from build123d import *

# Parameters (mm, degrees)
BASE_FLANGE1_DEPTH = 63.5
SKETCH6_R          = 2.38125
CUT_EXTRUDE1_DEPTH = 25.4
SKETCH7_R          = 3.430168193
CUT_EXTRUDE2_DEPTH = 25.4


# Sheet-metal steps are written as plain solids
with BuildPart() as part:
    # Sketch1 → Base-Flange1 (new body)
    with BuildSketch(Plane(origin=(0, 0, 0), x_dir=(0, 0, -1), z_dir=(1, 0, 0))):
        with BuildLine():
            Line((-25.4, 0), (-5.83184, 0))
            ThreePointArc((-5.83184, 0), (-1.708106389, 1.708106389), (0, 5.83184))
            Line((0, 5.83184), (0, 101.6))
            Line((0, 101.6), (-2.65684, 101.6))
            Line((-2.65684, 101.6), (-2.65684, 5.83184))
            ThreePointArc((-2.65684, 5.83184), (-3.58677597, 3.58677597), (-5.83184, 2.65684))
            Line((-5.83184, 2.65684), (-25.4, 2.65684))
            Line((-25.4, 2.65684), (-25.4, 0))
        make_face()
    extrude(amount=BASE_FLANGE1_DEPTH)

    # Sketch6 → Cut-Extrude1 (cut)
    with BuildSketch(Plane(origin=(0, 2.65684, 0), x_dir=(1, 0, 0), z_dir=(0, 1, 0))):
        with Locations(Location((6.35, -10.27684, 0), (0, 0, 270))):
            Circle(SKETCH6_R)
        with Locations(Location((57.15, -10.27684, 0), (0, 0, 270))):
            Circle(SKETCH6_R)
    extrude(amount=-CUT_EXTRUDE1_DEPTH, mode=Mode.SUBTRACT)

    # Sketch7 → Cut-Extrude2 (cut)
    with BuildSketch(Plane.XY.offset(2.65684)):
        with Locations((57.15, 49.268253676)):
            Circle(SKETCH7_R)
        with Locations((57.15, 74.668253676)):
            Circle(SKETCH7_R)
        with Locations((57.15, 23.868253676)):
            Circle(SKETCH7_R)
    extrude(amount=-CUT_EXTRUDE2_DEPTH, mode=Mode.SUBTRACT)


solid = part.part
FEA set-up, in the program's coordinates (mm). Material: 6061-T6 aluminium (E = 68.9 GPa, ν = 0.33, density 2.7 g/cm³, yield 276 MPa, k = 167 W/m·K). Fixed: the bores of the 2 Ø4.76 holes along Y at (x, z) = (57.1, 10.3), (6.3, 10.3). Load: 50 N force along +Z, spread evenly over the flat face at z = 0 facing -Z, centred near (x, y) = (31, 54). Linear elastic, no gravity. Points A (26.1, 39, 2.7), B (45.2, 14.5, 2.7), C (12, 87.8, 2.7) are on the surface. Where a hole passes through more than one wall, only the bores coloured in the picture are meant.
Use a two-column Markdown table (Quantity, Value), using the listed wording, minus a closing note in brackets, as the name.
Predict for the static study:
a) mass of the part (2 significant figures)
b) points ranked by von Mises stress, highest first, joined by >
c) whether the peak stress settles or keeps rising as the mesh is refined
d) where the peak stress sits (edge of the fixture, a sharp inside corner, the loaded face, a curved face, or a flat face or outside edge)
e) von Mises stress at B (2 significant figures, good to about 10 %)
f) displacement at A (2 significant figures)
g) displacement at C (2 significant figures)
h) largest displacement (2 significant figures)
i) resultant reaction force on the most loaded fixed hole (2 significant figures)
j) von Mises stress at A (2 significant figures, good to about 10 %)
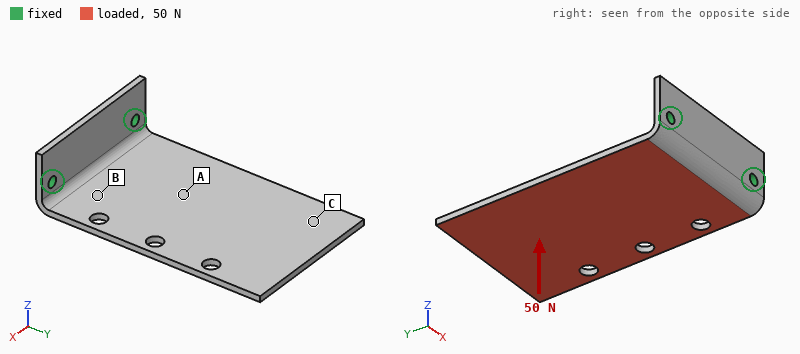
| Quantity | Value |
|---|---|
| mass of the part | 55 g |
| points ranked by von Mises stress, highest first, joined by > | B > A > C |
| whether the peak stress settles or keeps rising as the mesh is refined | keeps rising |
| where the peak stress sits | edge of the fixture |
| von Mises stress at B | 25 MPa |
| displacement at A | 0.32 mm |
| displacement at C | 1.0 mm |
| largest displacement | 1.3 mm |
| resultant reaction force on the most loaded fixed hole | 26 N |
| von Mises stress at A | 14 MPa |
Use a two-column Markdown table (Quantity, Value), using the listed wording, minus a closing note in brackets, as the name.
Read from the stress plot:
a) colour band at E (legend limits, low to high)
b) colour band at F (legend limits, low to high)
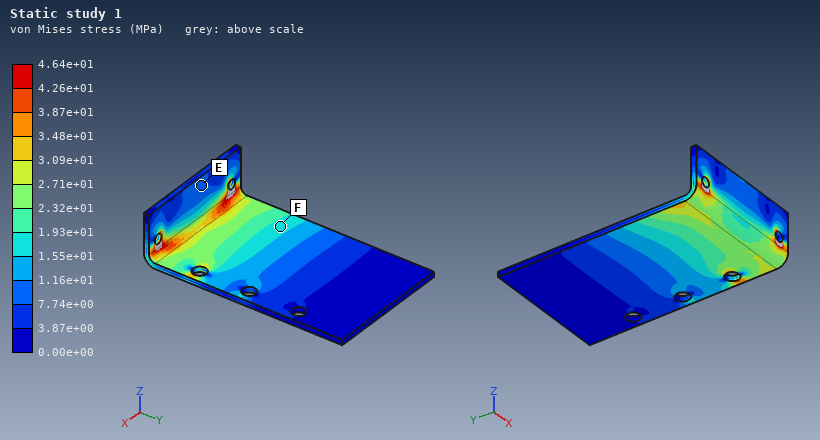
| Quantity | Value |
|---|---|
| colour band at E | 7.74e+00 to 1.16e+01 MPa |
| colour band at F | 1.55e+01 to 1.93e+01 MPa |
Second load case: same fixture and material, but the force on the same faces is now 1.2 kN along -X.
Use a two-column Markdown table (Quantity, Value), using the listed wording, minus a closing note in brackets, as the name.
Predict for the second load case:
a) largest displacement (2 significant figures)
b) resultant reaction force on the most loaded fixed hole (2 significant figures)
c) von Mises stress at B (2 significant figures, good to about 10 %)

| Quantity | Value |
|---|---|
| largest displacement | 0.40 mm |
| resultant reaction force on the most loaded fixed hole | 1.4 kN |
| von Mises stress at B | 47 MPa |
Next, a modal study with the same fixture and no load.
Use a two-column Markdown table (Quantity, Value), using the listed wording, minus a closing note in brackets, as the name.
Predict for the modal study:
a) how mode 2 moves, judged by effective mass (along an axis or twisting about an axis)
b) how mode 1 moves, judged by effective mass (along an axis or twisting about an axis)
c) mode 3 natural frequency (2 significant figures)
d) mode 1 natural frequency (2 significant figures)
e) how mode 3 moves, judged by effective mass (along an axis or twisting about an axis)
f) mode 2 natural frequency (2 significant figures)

| Quantity | Value |
|---|---|
| how mode 2 moves, judged by effective mass | twisting about Y |
| how mode 1 moves, judged by effective mass | along Z |
| mode 3 natural frequency | 1200 Hz |
| mode 1 natural frequency | 190 Hz |
| how mode 3 moves, judged by effective mass | along Z |
| mode 2 natural frequency | 720 Hz |
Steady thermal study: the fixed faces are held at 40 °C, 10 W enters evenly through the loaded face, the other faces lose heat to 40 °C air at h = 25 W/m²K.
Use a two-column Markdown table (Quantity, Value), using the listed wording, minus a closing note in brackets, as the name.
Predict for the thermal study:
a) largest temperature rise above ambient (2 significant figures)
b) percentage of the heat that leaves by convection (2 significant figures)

| Quantity | Value |
|---|---|
| largest temperature rise above ambient | 18 K |
| percentage of the heat that leaves by convection | 25 % |
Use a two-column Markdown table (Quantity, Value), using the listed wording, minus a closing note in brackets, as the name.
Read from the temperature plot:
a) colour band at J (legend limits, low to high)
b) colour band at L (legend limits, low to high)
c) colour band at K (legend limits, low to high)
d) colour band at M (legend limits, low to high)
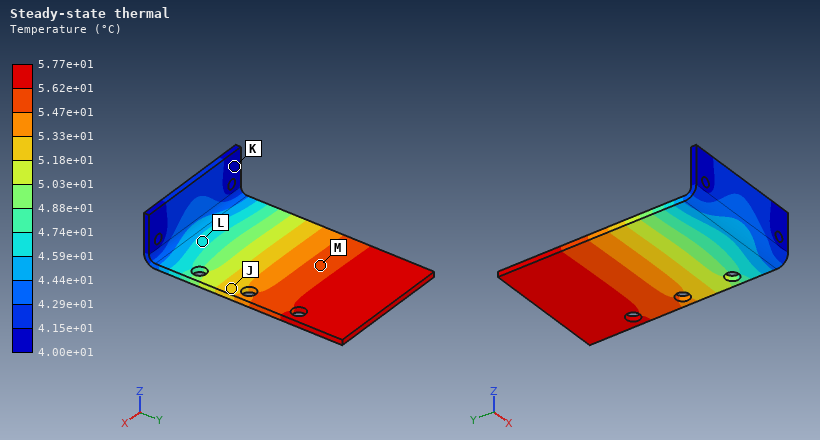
| Quantity | Value |
|---|---|
| colour band at J | 5.18e+01 to 5.33e+01 °C |
| colour band at L | 4.59e+01 to 4.74e+01 °C |
| colour band at K | 4.00e+01 to 4.15e+01 °C |
| colour band at M | 5.47e+01 to 5.62e+01 °C |
